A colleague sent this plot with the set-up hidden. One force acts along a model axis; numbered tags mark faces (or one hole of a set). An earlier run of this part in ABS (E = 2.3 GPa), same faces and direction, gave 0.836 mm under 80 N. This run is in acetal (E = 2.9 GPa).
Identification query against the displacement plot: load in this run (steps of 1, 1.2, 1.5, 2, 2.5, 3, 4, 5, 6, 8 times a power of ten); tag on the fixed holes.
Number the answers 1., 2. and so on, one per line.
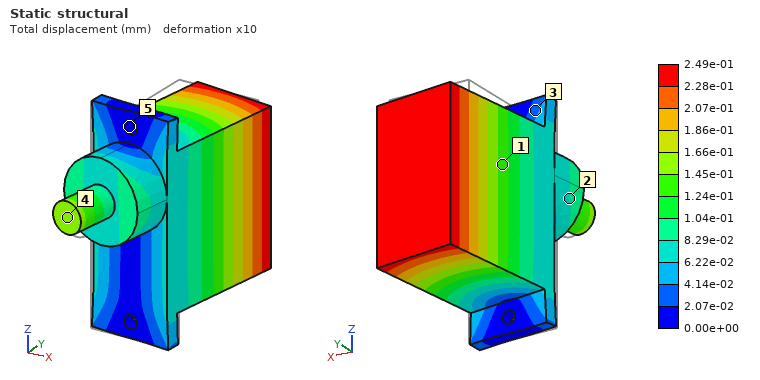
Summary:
1. 30 N
2. 5
